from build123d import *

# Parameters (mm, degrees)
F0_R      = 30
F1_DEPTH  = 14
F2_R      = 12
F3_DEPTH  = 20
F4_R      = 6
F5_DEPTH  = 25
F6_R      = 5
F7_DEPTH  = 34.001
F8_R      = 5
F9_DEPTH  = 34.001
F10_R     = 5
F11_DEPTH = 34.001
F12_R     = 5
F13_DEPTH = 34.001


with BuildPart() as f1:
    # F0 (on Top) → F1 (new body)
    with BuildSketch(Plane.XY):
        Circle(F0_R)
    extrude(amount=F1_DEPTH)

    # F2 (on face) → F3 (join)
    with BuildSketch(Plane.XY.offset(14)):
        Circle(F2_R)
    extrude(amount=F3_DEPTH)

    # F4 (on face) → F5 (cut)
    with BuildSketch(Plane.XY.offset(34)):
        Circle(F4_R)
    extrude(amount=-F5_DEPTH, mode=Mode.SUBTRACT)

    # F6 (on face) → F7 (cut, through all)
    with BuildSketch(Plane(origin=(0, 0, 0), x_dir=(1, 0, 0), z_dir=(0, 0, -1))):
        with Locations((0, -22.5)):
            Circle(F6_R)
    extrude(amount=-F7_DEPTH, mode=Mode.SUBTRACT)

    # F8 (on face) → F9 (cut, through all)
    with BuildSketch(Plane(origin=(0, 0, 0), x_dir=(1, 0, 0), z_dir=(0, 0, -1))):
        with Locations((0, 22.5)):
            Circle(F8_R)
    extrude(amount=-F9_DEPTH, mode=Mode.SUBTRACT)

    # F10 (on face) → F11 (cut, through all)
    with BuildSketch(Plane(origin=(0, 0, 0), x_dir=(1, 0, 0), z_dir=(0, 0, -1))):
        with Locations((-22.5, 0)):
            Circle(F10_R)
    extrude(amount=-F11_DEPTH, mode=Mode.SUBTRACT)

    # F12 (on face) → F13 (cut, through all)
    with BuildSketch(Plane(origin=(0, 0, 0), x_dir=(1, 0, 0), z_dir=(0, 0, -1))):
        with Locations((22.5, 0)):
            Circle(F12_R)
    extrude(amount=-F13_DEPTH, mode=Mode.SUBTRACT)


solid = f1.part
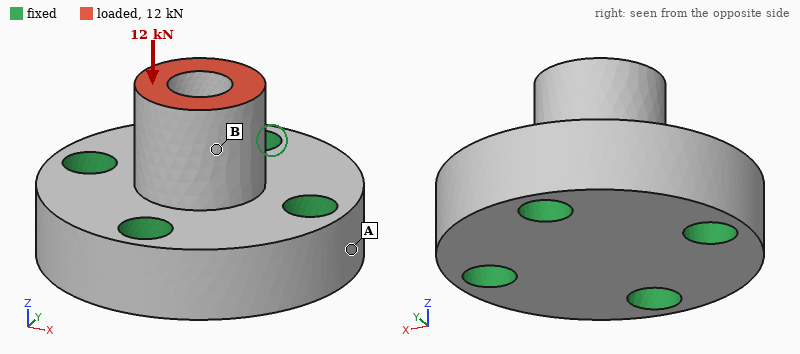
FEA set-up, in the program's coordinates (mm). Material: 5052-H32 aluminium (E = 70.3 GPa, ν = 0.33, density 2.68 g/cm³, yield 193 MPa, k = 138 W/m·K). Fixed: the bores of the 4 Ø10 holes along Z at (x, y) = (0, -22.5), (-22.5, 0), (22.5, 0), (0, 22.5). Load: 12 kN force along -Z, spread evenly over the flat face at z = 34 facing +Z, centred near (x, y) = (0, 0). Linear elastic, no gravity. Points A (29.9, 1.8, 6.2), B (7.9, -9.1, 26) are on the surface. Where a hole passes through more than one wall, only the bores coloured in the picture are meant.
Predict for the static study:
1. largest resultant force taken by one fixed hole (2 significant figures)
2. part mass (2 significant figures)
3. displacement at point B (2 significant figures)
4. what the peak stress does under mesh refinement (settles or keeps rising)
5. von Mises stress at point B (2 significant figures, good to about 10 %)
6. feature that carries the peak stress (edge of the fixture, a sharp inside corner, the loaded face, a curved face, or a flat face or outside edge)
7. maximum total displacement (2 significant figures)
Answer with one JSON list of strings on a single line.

["3.1 kN", "110 g", "13 µm", "keeps rising", "33 MPa", "edge of the fixture", "16 µm"]
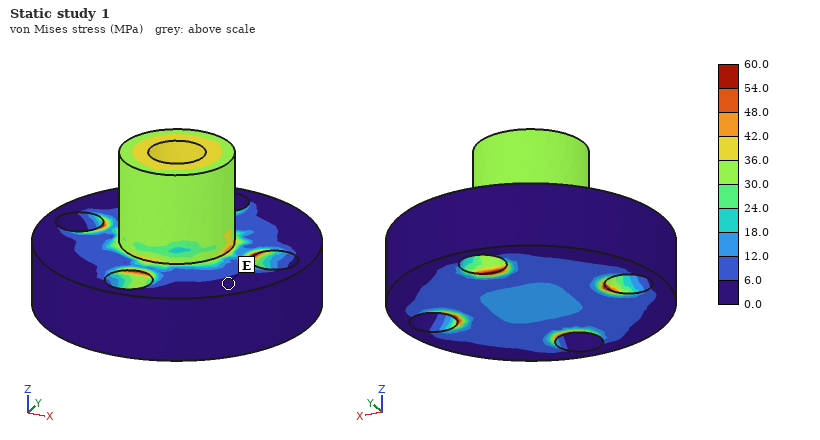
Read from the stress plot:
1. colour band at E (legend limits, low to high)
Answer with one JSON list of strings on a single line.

["0.0 to 6.0 MPa"]
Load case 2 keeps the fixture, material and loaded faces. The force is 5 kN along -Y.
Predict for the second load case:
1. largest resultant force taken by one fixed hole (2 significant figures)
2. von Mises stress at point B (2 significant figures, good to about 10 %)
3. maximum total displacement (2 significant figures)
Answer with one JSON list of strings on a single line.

["3.7 kN", "37 MPa", "53 µm"]
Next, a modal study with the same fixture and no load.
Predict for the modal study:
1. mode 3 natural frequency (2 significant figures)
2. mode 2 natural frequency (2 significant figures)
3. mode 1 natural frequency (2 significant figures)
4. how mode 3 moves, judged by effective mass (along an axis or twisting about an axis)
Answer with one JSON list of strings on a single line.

["33 kHz", "20 kHz", "20 kHz", "along Z"]
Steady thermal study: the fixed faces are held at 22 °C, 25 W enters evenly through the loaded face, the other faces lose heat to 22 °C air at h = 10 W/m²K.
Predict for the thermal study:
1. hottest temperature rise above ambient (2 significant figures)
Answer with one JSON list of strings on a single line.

["14 K"]
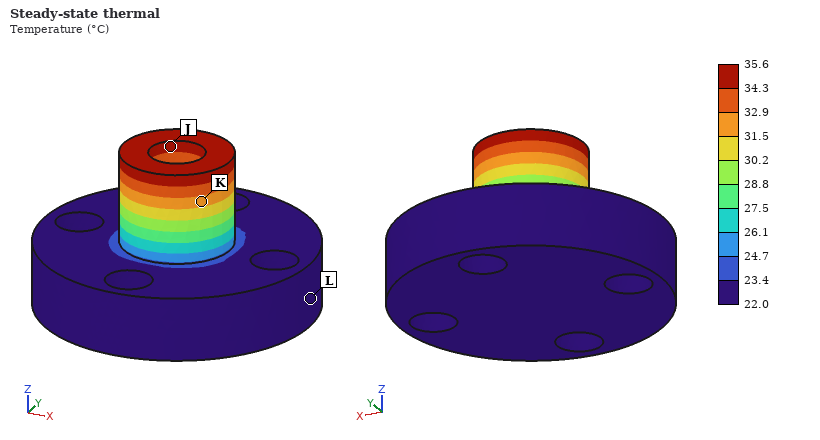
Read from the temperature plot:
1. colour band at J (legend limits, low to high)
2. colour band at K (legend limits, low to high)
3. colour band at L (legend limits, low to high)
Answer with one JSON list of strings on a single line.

["34.3 to 35.6 °C", "31.5 to 32.9 °C", "22.0 to 23.4 °C"]
